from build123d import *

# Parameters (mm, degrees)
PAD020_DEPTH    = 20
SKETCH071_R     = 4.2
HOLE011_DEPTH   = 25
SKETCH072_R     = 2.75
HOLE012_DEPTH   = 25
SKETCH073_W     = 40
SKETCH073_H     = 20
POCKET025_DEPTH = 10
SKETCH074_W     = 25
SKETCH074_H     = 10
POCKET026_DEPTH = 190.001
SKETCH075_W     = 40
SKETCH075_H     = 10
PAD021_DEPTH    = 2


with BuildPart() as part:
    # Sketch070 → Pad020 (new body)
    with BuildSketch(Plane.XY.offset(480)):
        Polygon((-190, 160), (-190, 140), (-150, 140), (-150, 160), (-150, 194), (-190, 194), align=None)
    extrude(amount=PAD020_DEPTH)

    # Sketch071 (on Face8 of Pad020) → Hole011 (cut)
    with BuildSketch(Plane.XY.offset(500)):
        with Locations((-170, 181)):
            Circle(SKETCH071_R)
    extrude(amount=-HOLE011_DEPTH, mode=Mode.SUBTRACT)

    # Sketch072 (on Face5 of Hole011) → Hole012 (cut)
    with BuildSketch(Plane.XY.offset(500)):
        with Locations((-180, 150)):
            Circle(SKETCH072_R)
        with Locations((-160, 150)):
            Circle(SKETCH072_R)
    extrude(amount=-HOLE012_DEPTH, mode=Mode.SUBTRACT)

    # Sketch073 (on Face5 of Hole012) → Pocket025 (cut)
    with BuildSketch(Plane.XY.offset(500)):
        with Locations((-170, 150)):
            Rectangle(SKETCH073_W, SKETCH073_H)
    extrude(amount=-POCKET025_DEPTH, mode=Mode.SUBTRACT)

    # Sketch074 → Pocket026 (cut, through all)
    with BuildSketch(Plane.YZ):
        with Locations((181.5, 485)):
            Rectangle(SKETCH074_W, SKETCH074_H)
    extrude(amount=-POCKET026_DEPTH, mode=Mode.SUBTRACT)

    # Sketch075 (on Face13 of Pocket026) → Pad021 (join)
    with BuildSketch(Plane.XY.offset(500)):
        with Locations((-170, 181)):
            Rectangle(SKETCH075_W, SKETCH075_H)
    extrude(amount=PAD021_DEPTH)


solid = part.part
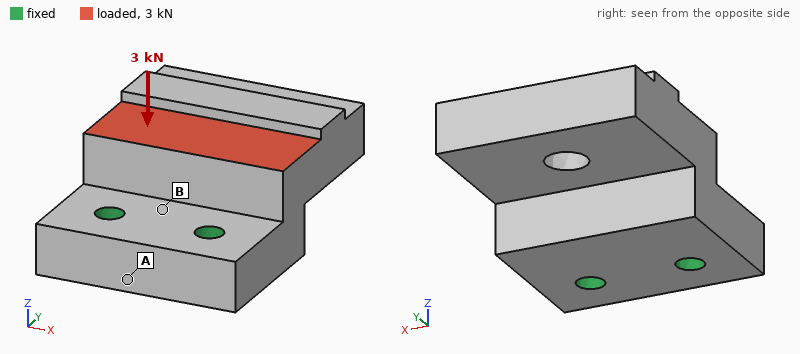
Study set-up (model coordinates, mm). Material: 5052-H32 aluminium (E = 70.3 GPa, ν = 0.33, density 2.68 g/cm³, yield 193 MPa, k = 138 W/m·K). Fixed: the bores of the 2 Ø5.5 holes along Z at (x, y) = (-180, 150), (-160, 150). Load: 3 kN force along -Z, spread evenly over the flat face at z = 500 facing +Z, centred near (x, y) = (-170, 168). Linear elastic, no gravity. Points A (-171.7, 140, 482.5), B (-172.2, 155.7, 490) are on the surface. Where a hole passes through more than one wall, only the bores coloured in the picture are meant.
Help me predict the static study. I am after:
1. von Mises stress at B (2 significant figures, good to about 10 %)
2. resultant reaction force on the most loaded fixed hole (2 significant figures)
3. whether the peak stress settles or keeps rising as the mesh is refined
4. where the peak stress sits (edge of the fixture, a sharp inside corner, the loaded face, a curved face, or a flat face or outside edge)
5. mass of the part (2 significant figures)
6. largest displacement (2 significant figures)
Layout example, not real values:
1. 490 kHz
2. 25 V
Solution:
1. 37 MPa
2. 1.5 kN
3. keeps rising
4. edge of the fixture
5. 67 g
6. 0.10 mm
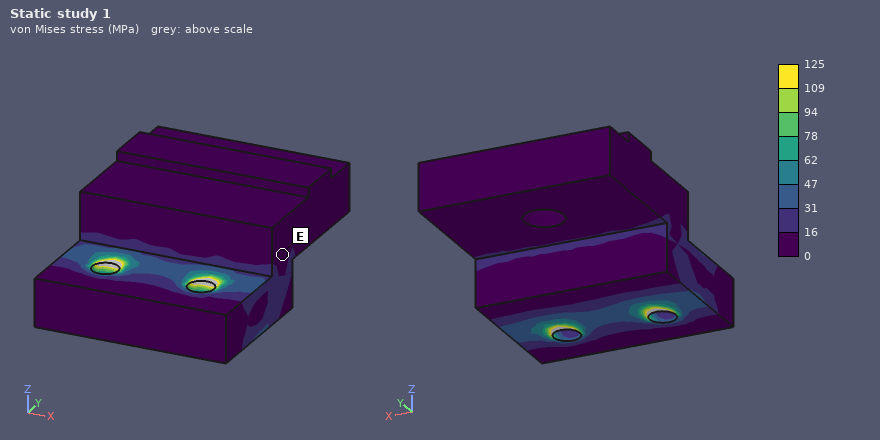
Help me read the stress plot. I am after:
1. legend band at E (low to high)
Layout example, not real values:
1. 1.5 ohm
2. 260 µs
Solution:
1. 0 to 16 MPa
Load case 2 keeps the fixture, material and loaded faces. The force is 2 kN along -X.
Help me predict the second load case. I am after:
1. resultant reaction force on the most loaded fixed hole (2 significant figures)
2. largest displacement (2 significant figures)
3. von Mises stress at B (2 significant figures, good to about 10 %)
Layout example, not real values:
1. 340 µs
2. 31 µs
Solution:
1. 2.0 kN
2. 21 µm
3. 27 MPa
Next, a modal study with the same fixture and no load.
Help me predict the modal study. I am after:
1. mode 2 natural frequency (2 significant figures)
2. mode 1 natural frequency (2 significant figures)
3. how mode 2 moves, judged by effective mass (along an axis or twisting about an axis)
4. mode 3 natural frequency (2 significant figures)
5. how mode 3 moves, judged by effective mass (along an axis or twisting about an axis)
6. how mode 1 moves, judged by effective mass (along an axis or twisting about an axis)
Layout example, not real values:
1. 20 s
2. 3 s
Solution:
1. 8300 Hz
2. 3600 Hz
3. along X
4. 9200 Hz
5. along X
6. along Z
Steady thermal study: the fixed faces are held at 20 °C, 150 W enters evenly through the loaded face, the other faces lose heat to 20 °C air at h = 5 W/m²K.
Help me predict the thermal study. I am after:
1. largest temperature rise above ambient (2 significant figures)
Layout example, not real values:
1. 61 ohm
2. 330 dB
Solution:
1. 66 K
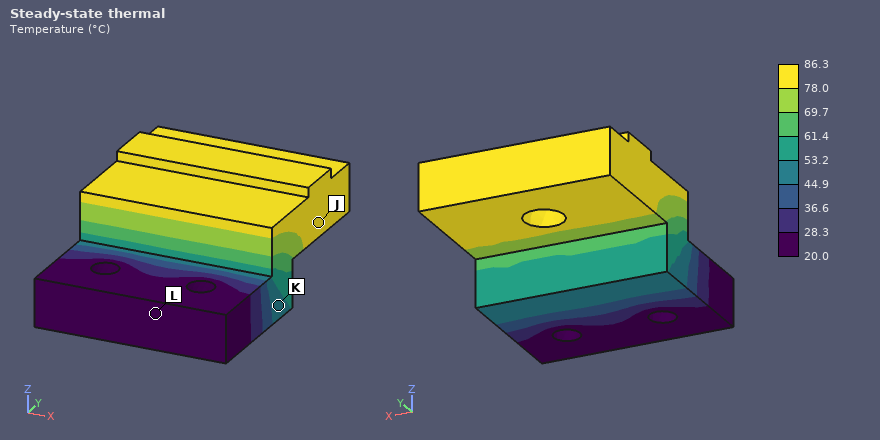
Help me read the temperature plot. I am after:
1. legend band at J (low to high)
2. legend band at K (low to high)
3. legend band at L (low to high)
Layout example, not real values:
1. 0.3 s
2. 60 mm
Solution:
1. 78.0 to 86.3 °C
2. 44.9 to 53.2 °C
3. 20.0 to 28.3 °C
